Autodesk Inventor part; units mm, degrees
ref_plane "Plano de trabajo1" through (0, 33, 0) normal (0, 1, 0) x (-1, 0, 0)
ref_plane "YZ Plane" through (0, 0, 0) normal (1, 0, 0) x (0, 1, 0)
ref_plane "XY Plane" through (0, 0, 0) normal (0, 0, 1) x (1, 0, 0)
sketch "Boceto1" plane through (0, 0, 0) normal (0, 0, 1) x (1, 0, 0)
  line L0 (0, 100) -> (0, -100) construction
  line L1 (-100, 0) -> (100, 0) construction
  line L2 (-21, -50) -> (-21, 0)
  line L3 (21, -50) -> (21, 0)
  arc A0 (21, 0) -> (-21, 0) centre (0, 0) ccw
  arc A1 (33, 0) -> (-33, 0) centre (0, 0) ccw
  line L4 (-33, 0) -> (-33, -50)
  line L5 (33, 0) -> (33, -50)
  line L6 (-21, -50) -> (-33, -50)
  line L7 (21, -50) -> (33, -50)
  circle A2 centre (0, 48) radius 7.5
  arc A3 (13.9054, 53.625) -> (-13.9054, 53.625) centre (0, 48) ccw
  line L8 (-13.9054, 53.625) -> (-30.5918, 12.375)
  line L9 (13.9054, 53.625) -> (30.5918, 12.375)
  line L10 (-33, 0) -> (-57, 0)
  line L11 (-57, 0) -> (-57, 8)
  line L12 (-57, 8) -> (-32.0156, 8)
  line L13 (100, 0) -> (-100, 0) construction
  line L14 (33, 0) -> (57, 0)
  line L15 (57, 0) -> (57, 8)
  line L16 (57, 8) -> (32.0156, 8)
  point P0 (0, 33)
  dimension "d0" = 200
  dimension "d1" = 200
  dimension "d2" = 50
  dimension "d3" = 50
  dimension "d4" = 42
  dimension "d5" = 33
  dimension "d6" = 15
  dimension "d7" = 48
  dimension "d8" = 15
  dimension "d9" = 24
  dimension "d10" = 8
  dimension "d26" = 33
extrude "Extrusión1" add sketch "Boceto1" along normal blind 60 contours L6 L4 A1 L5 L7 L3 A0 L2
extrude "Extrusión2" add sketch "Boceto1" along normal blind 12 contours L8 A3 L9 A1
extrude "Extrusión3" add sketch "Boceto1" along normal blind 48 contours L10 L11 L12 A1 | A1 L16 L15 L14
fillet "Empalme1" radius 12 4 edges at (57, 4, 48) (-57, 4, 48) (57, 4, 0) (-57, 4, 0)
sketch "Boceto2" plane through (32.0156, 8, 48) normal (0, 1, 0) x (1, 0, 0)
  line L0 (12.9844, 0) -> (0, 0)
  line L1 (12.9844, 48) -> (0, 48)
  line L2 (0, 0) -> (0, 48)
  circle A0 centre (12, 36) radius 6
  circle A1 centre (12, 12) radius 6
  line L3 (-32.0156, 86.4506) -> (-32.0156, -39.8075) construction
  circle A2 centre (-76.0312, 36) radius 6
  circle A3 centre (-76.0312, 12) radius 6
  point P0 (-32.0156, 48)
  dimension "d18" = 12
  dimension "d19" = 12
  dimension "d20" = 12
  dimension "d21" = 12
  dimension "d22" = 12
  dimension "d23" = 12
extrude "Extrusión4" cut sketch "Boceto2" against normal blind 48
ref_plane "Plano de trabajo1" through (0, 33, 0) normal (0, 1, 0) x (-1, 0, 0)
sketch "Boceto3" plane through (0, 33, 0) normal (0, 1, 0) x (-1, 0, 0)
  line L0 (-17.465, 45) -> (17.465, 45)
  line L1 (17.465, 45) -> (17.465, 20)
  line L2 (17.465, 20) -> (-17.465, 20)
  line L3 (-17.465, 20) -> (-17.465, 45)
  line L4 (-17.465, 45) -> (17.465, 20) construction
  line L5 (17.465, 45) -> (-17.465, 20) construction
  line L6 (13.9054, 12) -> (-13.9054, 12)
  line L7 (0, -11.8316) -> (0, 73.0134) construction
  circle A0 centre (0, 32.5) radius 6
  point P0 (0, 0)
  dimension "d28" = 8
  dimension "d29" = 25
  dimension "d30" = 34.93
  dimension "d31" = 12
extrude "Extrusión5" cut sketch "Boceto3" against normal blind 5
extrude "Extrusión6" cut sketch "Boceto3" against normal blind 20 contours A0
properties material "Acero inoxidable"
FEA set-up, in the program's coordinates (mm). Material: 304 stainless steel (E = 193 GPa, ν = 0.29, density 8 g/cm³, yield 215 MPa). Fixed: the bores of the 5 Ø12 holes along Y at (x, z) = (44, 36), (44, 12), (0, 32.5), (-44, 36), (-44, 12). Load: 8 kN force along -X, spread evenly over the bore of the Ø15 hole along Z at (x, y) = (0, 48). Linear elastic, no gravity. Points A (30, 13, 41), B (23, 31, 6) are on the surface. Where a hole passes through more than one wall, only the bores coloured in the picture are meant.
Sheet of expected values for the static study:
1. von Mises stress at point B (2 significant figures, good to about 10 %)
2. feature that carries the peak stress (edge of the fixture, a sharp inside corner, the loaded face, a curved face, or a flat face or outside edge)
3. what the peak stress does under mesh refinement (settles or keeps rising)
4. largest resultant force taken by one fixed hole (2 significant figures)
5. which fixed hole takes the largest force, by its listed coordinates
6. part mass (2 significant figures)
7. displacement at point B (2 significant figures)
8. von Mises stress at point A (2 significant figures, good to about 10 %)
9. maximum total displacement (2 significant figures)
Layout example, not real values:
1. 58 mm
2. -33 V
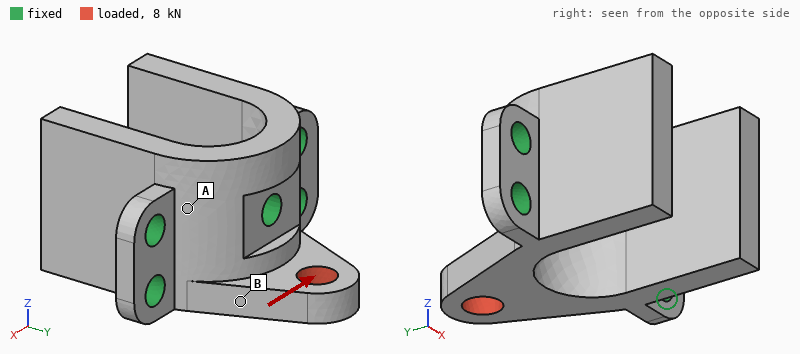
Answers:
1. 49 MPa
2. edge of the fixture
3. keeps rising
4. 4.1 kN
5. (0, 32.5)
6. 1.2 kg
7. 9.6 µm
8. 8.4 MPa
9. 28 µm
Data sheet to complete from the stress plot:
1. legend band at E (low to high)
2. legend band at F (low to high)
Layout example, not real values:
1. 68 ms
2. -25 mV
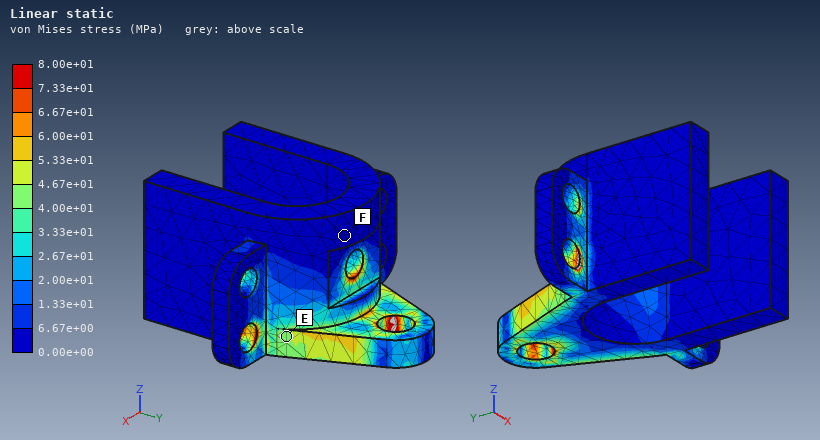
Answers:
1. 4.00e+01 to 4.67e+01 MPa
2. 0.00e+00 to 6.67e+00 MPa
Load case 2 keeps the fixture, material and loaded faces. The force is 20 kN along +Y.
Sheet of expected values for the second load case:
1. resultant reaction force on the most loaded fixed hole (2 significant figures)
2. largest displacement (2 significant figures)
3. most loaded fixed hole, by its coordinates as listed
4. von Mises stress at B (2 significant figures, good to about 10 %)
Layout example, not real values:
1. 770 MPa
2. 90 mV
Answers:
1. 11 kN
2. 50 µm
3. (0, 32.5)
4. 55 MPa
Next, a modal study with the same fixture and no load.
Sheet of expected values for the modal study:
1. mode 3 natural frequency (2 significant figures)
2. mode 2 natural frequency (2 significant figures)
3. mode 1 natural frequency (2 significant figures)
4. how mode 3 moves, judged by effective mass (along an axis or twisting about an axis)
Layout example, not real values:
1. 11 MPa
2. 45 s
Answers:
1. 4400 Hz
2. 2700 Hz
3. 2700 Hz
4. along Z
